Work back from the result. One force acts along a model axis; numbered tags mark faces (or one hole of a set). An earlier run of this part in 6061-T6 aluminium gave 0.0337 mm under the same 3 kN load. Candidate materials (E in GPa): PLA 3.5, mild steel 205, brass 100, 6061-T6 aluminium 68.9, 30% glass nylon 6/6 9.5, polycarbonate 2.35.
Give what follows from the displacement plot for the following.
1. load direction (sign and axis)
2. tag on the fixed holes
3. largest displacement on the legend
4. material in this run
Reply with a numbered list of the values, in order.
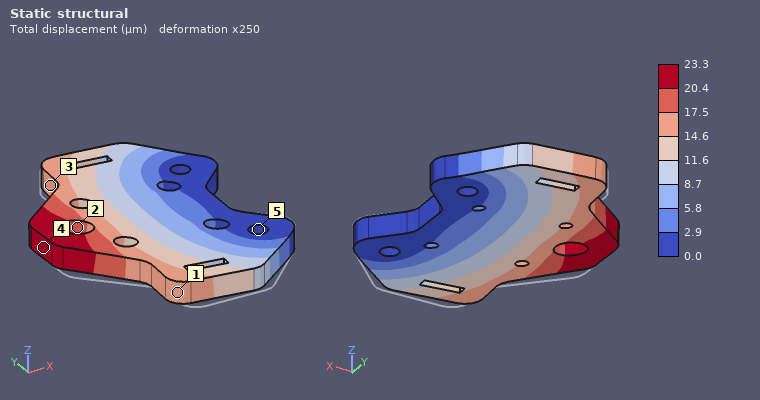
1. +Y
2. 5
3. 23.3 µm
4. brass
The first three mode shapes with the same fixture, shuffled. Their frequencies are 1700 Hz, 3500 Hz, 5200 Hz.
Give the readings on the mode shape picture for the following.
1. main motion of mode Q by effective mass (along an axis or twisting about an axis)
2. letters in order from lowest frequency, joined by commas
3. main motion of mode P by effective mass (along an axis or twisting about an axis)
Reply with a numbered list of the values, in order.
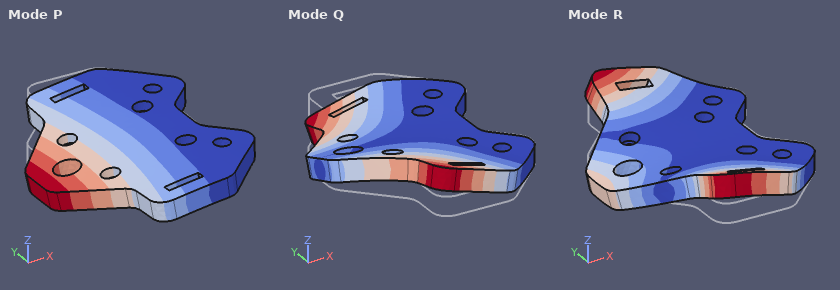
1. twisting about X
2. P, Q, R
3. along Z
